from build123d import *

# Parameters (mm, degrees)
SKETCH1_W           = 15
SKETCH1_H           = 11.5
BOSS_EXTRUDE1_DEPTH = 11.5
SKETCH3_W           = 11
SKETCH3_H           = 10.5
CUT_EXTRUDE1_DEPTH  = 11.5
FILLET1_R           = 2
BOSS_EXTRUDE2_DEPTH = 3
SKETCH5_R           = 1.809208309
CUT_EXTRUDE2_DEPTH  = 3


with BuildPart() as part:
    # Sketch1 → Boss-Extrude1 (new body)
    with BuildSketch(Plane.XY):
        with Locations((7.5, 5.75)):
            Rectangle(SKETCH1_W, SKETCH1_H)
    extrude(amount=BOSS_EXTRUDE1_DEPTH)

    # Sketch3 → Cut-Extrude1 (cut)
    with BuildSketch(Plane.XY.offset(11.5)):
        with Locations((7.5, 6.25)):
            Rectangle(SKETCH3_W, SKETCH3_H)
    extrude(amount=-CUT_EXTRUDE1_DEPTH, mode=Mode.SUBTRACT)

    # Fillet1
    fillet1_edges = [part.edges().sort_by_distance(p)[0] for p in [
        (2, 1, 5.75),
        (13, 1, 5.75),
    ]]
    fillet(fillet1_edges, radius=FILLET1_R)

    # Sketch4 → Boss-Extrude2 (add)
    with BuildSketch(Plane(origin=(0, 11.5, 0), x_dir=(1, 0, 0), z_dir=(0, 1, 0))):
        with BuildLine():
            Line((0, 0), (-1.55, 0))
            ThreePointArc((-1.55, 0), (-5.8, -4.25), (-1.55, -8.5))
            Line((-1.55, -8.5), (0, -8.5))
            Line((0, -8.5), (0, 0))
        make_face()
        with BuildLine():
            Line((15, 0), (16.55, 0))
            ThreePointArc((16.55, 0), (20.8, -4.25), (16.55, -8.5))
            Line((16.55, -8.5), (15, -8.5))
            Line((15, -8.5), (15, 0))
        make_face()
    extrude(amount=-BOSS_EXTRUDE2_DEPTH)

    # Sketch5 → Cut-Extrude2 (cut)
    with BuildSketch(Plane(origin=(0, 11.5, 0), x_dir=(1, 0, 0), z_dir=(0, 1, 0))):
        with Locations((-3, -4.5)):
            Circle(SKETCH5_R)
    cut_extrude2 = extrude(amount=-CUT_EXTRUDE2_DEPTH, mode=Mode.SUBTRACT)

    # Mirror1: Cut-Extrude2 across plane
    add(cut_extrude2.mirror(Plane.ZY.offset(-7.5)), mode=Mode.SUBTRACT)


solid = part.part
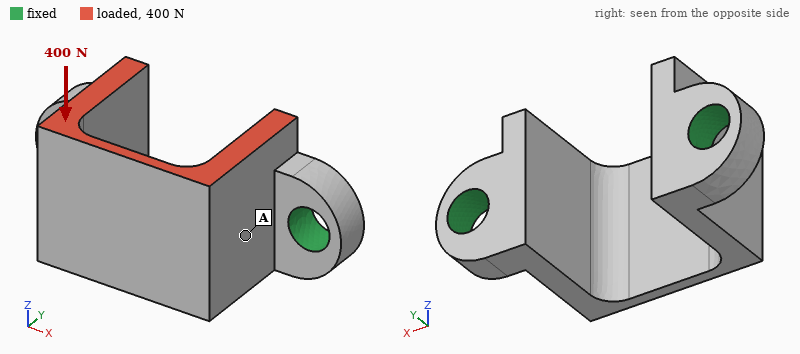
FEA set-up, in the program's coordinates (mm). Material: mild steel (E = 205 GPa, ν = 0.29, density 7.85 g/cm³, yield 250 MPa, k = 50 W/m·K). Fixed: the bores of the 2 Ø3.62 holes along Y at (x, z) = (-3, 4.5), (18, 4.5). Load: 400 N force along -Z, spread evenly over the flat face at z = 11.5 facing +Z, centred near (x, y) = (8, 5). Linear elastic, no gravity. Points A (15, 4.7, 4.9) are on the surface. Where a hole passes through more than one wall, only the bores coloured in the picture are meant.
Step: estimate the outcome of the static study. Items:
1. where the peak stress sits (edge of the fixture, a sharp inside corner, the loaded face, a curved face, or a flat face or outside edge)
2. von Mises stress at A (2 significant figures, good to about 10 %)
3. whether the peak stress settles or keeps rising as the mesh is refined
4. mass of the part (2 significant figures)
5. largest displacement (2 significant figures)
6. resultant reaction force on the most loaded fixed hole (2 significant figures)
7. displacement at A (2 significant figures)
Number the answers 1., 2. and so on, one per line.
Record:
1. edge of the fixture
2. 13 MPa
3. keeps rising
4. 6.8 g
5. 7.9 µm
6. 200 N
7. 3.6 µm
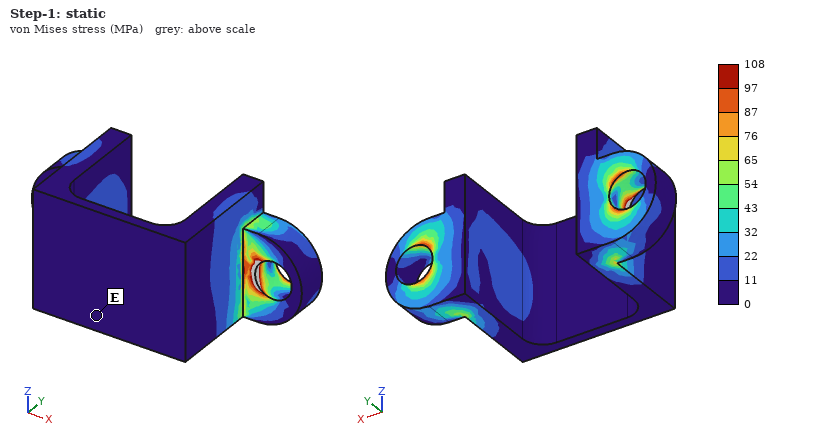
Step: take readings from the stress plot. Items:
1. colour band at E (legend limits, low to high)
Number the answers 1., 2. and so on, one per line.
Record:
1. 0 to 11 MPa
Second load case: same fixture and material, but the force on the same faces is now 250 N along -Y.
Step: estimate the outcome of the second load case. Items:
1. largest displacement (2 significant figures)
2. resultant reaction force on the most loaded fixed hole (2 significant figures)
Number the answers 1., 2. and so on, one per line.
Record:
1. 9.0 µm
2. 130 N
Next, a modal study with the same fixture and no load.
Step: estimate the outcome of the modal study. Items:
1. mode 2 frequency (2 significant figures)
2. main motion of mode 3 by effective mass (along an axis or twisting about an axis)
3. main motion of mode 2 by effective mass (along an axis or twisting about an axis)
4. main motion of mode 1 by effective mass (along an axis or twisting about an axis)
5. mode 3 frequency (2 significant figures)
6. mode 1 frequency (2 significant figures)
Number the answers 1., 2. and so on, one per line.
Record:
1. 18 kHz
2. twisting about Y
3. along Z
4. along X
5. 21 kHz
6. 14 kHz
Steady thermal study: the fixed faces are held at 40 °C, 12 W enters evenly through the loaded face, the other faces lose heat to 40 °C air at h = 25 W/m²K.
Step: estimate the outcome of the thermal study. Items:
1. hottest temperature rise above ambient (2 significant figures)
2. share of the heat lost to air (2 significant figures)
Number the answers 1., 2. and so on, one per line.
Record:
1. 59 K
2. 5.8 %
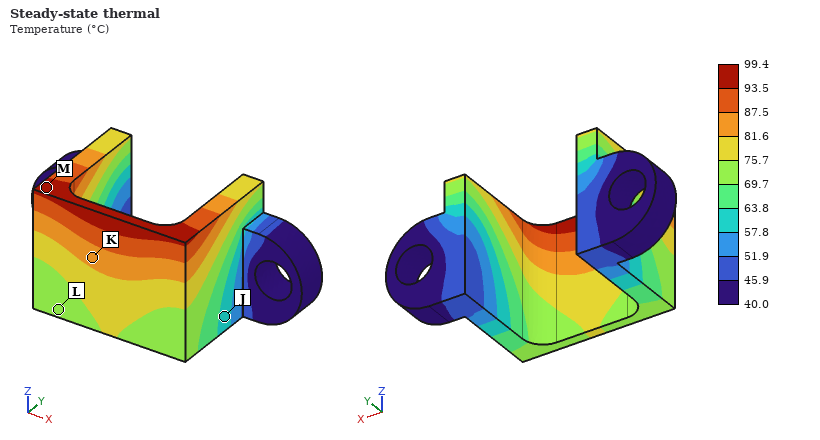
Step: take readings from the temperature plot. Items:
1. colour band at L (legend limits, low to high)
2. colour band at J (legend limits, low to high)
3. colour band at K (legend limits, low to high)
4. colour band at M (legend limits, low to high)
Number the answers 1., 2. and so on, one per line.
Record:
1. 69.7 to 75.7 °C
2. 57.8 to 63.8 °C
3. 81.6 to 87.5 °C
4. 93.5 to 99.4 °C
